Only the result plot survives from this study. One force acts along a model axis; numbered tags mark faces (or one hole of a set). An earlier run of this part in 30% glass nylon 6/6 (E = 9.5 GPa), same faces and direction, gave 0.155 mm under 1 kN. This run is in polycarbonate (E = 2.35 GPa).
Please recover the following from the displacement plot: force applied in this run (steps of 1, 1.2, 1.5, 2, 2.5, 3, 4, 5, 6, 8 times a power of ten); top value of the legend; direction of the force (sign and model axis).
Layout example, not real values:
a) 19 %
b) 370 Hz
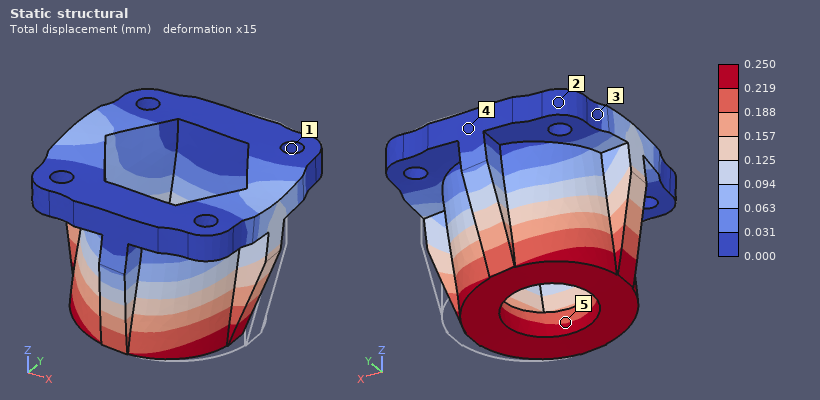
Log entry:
a) 400 N
b) 0.250 mm
c) -X
